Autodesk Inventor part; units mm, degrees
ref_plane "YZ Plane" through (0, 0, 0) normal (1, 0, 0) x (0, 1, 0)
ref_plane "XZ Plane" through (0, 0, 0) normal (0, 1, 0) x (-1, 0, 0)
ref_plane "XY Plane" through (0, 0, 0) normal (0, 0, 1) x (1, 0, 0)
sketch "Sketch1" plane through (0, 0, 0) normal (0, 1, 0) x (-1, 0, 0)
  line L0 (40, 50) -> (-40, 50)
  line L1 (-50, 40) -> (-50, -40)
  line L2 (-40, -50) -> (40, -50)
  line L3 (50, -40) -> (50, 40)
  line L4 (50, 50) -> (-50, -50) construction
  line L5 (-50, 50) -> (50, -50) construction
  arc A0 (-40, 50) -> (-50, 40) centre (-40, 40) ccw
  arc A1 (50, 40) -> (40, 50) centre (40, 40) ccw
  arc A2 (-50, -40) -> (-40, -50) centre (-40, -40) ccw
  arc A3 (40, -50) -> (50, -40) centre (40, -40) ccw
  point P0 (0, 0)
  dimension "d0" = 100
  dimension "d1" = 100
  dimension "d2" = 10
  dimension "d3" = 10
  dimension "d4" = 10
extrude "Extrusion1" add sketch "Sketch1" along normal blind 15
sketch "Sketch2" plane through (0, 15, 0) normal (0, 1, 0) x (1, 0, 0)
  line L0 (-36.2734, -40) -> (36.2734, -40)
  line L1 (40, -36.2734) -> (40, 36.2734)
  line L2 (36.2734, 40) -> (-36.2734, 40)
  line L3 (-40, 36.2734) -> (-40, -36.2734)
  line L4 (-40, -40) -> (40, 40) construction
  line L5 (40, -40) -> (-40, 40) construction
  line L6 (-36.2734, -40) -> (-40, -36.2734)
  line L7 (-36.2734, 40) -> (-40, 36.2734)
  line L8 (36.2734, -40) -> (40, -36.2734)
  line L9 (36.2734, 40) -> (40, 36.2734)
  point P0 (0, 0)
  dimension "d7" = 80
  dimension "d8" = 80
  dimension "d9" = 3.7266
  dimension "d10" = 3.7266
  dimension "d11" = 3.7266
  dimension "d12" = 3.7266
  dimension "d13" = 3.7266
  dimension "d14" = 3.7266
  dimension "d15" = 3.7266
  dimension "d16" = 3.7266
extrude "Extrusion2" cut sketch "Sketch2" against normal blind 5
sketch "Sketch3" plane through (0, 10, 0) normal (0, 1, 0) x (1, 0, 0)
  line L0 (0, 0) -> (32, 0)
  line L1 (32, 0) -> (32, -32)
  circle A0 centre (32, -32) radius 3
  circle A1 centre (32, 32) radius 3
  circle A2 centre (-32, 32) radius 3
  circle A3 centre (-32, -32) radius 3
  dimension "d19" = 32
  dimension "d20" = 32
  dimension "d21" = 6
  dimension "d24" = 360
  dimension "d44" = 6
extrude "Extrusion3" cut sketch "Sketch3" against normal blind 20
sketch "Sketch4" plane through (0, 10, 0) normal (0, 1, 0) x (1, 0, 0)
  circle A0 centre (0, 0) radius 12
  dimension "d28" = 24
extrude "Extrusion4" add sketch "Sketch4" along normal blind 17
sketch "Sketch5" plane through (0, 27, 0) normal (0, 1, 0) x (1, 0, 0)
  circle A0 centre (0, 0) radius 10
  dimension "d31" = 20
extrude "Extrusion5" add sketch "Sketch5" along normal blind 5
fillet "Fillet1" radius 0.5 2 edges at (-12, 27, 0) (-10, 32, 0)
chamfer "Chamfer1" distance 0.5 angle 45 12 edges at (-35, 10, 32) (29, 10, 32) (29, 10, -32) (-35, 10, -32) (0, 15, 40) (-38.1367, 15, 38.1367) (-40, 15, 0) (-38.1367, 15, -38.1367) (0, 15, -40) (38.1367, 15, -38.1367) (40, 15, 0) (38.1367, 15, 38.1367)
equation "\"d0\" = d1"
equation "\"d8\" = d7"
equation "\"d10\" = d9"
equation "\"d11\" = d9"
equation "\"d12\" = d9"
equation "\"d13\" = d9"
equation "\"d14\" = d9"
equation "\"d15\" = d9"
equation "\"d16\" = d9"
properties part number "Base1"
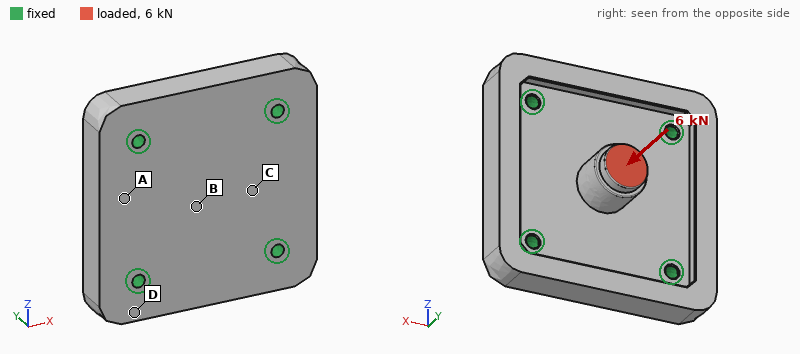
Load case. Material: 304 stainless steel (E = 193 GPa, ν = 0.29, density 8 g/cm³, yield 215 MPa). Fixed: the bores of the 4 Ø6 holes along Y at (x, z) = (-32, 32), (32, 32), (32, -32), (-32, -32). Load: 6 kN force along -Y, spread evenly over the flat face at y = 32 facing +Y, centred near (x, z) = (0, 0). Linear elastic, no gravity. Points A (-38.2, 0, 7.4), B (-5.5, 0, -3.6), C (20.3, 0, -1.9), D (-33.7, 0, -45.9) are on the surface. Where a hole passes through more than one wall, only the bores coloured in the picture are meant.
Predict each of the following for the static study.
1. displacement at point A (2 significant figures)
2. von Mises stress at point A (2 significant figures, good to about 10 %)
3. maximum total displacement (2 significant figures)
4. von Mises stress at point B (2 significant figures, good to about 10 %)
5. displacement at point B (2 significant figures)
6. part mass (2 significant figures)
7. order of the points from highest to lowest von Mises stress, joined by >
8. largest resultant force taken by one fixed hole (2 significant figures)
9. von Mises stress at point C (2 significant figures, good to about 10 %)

3.3 µm
13 MPa
16 µm
31 MPa
14 µm
1000 g
B > C > A > D
1.5 kN
22 MPa
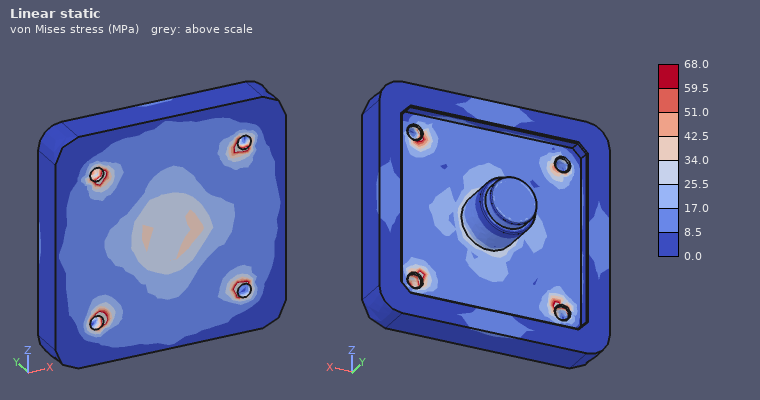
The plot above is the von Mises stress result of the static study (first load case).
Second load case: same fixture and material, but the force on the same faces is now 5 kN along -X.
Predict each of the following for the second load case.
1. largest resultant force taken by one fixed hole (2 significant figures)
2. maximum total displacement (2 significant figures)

1.8 kN
31 µm
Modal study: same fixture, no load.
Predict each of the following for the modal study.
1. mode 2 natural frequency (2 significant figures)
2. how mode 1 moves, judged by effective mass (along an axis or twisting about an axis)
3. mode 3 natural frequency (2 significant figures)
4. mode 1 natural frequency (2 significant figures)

8900 Hz
along Y
9300 Hz
6800 Hz
